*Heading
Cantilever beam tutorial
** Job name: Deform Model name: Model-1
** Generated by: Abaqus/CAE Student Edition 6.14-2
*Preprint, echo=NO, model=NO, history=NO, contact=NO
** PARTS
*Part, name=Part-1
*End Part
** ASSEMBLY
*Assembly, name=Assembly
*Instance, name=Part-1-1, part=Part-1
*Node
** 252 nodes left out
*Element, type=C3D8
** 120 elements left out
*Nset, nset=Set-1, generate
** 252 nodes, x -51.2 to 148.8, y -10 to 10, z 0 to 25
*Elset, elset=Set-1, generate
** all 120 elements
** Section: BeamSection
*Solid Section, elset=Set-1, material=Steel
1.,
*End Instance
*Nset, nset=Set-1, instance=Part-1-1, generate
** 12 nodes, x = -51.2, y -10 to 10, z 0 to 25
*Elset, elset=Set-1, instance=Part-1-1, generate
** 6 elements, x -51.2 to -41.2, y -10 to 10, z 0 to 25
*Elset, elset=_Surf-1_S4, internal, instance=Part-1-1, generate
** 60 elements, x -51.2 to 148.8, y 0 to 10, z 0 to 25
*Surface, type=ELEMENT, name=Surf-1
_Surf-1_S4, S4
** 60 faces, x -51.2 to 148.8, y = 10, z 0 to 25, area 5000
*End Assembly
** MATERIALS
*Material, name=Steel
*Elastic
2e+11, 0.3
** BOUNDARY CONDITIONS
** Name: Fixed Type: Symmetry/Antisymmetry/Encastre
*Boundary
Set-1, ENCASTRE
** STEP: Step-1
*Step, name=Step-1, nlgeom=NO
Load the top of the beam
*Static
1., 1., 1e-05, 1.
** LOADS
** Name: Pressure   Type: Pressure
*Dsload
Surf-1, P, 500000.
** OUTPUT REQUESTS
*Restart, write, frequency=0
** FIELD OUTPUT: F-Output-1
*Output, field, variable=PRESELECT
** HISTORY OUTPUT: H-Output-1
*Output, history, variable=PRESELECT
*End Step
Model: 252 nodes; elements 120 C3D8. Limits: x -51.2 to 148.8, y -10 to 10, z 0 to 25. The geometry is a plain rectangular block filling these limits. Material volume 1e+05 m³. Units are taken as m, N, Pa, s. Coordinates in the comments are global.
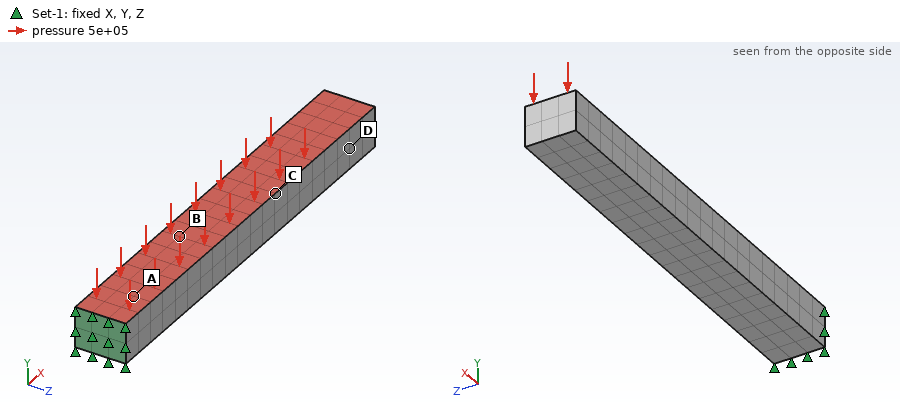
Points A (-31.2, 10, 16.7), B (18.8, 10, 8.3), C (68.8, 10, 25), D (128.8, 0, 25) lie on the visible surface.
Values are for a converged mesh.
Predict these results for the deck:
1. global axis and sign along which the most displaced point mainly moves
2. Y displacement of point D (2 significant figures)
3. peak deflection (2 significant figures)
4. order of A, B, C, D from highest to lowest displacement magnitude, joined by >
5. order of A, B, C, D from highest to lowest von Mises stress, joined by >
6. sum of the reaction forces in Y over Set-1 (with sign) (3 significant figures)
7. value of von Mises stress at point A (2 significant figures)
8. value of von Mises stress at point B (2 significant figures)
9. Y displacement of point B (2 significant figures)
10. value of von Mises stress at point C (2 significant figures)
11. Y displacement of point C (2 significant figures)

-Y
-0.65 m
0.75 m
D > C > B > A
A > B > C > D
2.50e+09 N
1.2e+08 Pa
6.4e+07 Pa
-0.15 m
2.4e+07 Pa
-0.36 m
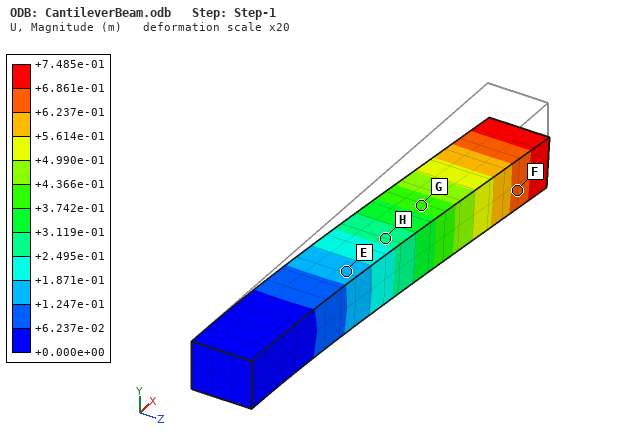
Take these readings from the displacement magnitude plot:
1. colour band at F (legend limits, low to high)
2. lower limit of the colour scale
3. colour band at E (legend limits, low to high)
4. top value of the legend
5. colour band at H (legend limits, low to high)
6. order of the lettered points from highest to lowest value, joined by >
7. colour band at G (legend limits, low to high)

+6.237e-01 to +6.861e-01 m
+0.000e+00 m
+1.247e-01 to +1.871e-01 m
+7.485e-01 m
+2.495e-01 to +3.119e-01 m
F > G > H > E
+3.742e-01 to +4.366e-01 m
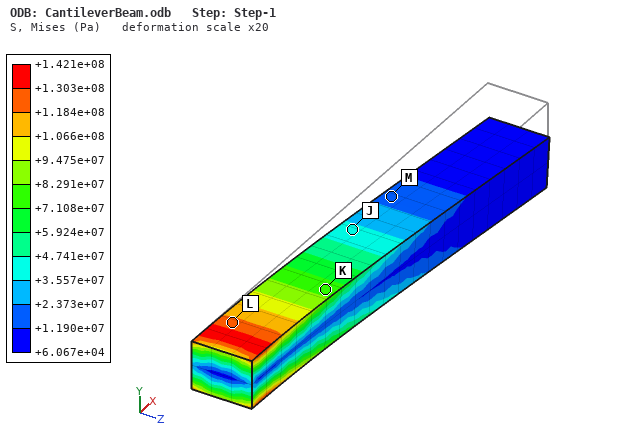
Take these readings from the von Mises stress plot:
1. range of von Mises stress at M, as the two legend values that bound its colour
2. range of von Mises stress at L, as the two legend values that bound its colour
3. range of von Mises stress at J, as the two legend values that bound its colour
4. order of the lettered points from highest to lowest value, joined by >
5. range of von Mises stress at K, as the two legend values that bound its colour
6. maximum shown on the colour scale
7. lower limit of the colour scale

+1.190e+07 to +2.373e+07 Pa
+1.184e+08 to +1.303e+08 Pa
+3.557e+07 to +4.741e+07 Pa
L > K > J > M
+7.108e+07 to +8.291e+07 Pa
+1.421e+08 Pa
+6.067e+04 Pa
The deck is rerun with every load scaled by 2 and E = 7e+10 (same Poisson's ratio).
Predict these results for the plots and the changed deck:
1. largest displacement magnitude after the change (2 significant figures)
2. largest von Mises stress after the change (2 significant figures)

4.3 m
2.8e+08 Pa
